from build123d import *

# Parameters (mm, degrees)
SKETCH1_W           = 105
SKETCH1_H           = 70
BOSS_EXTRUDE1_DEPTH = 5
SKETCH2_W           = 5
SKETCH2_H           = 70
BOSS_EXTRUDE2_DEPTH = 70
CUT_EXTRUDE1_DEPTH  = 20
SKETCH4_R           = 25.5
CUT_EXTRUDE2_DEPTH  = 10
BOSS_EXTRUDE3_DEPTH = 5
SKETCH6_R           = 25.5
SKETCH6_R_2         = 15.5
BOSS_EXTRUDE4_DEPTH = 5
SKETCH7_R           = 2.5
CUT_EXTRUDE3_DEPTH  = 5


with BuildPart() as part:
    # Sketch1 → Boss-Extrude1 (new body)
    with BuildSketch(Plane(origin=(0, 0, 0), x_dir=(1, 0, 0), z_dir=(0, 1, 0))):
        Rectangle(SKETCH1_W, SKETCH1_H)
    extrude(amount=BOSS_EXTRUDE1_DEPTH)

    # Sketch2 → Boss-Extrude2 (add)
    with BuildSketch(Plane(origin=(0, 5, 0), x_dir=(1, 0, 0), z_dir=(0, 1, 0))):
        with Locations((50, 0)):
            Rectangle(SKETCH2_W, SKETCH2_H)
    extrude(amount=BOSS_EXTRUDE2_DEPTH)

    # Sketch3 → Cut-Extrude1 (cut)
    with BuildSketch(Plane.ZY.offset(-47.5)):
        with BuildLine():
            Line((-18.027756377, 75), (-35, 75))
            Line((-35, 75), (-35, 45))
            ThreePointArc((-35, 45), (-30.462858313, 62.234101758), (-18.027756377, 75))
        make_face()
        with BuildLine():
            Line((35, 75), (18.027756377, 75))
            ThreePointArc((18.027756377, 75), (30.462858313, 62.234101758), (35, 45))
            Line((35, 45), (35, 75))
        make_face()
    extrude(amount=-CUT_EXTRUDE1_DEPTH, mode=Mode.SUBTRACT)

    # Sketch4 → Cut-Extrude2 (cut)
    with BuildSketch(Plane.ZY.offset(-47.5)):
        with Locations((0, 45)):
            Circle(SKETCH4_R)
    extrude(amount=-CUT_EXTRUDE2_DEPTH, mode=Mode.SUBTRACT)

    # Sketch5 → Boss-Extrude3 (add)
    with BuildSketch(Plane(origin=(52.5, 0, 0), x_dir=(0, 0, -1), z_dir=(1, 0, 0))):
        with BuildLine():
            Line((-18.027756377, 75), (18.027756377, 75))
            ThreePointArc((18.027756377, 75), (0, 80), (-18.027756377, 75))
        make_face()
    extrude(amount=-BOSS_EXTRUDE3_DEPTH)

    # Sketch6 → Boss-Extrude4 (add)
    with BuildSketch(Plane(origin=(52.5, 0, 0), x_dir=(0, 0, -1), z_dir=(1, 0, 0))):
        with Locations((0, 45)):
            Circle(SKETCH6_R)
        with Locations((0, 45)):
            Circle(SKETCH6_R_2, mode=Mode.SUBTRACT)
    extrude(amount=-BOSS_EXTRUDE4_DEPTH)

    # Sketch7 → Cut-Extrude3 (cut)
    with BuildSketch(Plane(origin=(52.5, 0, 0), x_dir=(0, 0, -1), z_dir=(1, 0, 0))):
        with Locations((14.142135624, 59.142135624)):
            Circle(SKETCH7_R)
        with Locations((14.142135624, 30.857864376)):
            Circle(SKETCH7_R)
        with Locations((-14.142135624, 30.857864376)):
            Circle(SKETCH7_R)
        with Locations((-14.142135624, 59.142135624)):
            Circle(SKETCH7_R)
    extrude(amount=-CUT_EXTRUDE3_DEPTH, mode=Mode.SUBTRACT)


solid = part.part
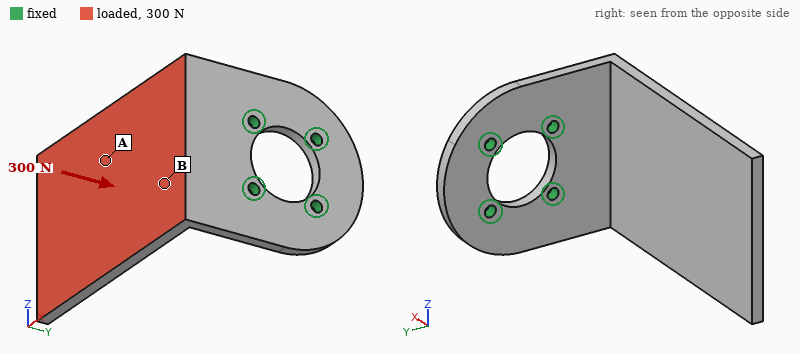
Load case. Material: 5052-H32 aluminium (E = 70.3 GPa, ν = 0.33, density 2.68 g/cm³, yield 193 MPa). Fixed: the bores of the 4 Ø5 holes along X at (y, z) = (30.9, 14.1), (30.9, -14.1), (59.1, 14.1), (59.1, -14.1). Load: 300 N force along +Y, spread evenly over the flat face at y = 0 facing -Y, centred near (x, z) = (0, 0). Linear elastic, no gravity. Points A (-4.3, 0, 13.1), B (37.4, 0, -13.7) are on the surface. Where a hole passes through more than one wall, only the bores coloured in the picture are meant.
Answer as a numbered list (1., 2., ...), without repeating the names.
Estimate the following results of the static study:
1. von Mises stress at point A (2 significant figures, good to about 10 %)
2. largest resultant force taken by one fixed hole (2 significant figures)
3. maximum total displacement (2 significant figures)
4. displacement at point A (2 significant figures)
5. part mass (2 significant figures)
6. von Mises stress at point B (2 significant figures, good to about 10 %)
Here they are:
1. 11 MPa
2. 170 N
3. 1.5 mm
4. 0.73 mm
5. 150 g
6. 35 MPa
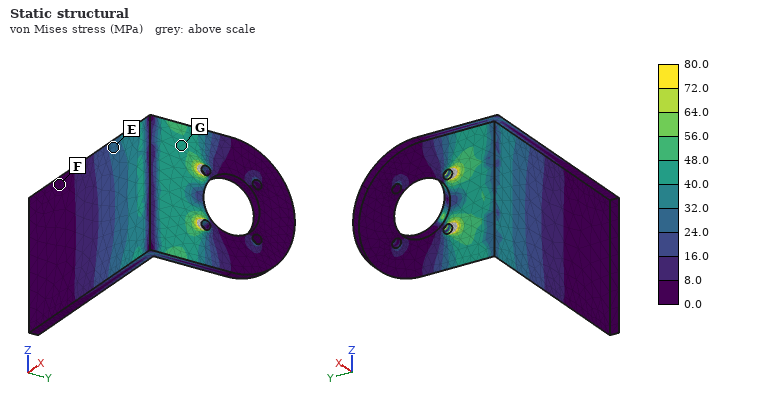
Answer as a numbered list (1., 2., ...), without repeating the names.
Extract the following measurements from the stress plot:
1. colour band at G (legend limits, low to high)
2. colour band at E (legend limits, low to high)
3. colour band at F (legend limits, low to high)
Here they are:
1. 40.0 to 48.0 MPa
2. 24.0 to 32.0 MPa
3. 0.0 to 8.0 MPa
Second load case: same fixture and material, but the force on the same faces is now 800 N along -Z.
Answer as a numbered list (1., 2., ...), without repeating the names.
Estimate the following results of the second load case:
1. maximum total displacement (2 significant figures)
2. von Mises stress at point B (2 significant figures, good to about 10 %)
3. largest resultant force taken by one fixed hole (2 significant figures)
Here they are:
1. 0.72 mm
2. 19 MPa
3. 1.3 kN
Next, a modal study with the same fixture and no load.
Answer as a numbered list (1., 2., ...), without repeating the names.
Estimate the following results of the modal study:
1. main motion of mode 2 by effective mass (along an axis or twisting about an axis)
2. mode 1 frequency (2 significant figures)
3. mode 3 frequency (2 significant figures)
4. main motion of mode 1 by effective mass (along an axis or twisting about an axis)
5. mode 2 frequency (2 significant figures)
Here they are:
1. along Z
2. 270 Hz
3. 1200 Hz
4. along Y
5. 620 Hz
